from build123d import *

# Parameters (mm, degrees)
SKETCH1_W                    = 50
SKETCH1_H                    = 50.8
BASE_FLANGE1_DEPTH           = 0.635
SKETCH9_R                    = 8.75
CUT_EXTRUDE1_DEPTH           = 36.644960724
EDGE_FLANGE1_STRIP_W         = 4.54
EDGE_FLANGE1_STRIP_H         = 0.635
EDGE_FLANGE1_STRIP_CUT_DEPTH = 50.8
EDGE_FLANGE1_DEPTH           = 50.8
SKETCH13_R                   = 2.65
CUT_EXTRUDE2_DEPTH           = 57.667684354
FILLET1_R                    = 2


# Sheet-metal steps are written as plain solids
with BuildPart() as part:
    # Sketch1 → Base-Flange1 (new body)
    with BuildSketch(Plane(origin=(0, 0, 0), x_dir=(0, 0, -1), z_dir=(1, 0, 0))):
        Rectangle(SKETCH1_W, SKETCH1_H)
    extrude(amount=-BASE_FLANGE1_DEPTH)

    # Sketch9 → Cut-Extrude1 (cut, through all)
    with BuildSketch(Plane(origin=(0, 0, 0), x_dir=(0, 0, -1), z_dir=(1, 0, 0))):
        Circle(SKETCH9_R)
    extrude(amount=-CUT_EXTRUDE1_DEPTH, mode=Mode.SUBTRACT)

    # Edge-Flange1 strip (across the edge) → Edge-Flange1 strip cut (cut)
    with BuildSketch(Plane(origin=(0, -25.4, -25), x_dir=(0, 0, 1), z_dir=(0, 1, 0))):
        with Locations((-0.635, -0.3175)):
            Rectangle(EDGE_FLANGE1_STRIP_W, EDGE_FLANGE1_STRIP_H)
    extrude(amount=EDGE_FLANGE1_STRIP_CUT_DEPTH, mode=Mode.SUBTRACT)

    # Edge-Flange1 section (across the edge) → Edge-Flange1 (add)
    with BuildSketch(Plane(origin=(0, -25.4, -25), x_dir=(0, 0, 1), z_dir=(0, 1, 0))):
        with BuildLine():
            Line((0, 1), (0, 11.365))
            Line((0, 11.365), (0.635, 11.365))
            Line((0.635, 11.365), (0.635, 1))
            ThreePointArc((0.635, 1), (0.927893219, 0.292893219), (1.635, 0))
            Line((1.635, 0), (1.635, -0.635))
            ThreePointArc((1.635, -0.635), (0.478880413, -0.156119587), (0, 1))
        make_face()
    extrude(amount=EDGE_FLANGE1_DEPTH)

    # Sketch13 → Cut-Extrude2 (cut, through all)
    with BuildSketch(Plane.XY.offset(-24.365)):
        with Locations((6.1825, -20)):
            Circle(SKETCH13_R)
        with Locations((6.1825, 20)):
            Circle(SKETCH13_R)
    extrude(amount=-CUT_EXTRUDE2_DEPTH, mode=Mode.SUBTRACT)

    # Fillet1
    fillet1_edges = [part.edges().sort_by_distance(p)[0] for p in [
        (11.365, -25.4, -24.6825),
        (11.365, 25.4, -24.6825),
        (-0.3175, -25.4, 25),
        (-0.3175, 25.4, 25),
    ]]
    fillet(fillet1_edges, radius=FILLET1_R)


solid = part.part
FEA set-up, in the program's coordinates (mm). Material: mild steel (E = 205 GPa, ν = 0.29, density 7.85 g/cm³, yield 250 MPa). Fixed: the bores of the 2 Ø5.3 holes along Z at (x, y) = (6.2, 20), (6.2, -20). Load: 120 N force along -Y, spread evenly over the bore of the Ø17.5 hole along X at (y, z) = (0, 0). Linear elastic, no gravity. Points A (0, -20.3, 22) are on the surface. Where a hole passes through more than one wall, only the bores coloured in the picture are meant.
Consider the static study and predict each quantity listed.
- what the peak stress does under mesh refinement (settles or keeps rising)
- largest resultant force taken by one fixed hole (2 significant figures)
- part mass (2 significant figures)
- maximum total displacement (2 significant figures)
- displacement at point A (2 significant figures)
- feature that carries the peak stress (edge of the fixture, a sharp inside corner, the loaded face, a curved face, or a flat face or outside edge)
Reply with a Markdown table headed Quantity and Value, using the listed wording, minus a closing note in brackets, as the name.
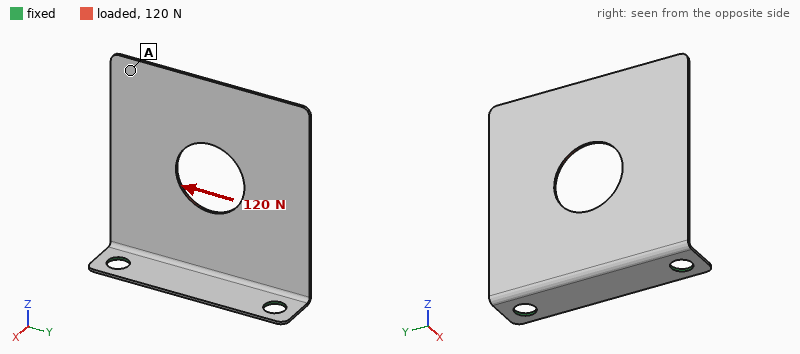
| Quantity | Value |
|---|---|
| what the peak stress does under mesh refinement | keeps rising |
| largest resultant force taken by one fixed hole | 96 N |
| part mass | 14 g |
| maximum total displacement | 0.17 mm |
| displacement at point A | 0.15 mm |
| feature that carries the peak stress | edge of the fixture |
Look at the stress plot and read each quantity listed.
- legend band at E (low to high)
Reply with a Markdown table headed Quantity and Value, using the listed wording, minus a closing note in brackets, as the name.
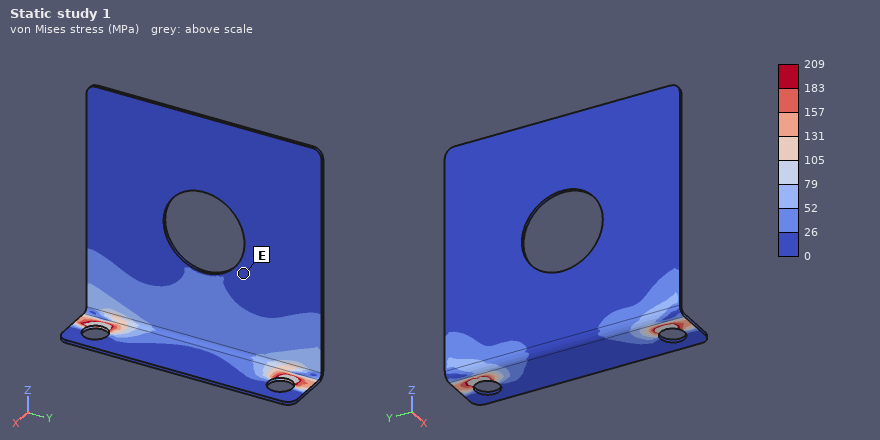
| Quantity | Value |
|---|---|
| legend band at E | 0 to 26 MPa |
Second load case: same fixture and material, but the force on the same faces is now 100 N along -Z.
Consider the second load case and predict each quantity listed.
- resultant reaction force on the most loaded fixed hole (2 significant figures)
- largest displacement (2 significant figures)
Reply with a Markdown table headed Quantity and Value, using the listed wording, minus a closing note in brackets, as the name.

| Quantity | Value |
|---|---|
| resultant reaction force on the most loaded fixed hole | 51 N |
| largest displacement | 0.32 mm |
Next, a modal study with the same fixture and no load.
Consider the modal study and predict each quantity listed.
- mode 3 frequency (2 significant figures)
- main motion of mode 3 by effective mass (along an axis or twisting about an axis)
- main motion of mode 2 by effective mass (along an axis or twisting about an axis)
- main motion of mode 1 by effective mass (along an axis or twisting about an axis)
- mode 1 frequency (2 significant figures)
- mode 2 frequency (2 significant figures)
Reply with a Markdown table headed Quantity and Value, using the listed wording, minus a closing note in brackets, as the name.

| Quantity | Value |
|---|---|
| mode 3 frequency | 1100 Hz |
| main motion of mode 3 by effective mass | along X |
| main motion of mode 2 by effective mass | twisting about Z |
| main motion of mode 1 by effective mass | along X |
| mode 1 frequency | 180 Hz |
| mode 2 frequency | 460 Hz |
